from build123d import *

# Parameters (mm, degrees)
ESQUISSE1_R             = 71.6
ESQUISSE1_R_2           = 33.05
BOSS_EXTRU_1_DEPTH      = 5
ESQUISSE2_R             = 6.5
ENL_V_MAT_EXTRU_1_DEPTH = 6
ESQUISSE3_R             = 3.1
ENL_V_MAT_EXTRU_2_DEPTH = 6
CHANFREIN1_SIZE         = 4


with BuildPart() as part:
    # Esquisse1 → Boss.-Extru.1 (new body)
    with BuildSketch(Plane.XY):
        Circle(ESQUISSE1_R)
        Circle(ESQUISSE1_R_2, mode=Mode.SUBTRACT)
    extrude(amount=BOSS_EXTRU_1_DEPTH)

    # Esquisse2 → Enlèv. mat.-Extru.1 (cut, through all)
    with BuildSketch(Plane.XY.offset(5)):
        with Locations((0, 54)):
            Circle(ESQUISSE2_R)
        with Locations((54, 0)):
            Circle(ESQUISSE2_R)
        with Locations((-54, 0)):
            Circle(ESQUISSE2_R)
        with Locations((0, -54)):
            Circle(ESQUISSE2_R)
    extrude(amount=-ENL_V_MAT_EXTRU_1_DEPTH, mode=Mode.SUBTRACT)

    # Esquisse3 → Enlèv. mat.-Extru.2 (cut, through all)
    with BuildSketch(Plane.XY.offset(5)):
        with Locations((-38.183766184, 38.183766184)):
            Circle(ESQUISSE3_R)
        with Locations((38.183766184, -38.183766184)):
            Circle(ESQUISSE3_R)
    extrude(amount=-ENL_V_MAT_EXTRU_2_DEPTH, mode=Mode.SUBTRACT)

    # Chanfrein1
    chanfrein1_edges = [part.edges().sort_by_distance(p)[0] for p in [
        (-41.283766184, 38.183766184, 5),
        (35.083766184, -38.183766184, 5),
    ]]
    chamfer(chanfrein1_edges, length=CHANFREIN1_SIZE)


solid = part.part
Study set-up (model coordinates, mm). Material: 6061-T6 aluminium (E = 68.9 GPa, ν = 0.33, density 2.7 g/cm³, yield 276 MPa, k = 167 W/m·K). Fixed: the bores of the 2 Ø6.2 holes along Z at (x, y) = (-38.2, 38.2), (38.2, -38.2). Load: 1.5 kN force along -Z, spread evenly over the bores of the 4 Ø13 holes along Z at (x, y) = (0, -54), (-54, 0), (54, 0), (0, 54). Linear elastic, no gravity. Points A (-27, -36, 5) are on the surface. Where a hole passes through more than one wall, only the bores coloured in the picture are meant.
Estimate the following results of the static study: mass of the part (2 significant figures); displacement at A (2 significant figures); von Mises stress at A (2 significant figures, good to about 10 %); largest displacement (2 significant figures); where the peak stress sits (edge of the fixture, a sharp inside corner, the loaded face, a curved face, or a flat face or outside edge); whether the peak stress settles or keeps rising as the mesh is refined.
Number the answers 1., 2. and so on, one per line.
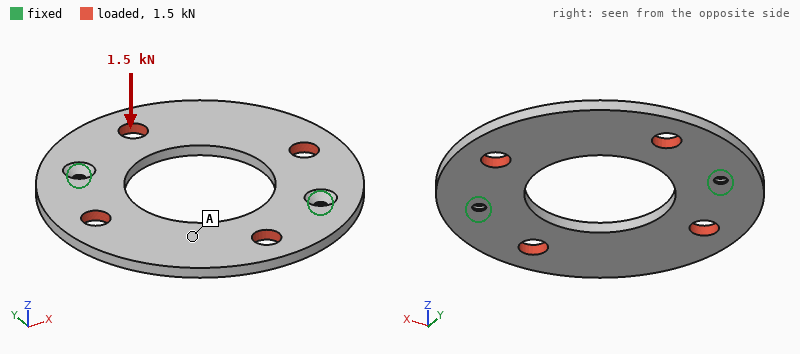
1. 160 g
2. 0.50 mm
3. 21 MPa
4. 0.79 mm
5. edge of the fixture
6. keeps rising
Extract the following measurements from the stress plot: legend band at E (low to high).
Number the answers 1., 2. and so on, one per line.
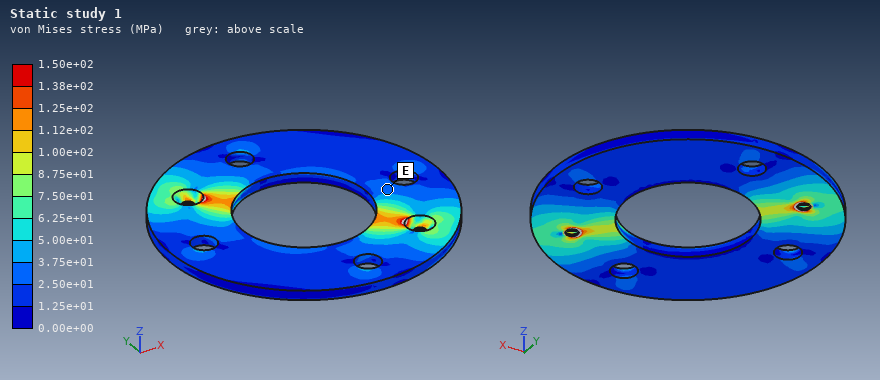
1. 2.50e+01 to 3.75e+01 MPa
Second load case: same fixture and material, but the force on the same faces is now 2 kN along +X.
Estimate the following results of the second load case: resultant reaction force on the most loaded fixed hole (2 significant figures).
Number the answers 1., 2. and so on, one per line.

1. 1.0 kN
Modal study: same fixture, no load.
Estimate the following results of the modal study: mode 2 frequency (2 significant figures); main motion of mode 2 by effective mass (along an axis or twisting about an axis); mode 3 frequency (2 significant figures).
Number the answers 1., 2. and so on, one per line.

1. 680 Hz
2. along Z
3. 1300 Hz
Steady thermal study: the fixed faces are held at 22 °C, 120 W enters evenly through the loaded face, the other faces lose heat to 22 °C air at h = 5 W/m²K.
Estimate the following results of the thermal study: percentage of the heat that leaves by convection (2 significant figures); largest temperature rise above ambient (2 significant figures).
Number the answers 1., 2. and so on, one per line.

1. 5.9 %
2. 67 K
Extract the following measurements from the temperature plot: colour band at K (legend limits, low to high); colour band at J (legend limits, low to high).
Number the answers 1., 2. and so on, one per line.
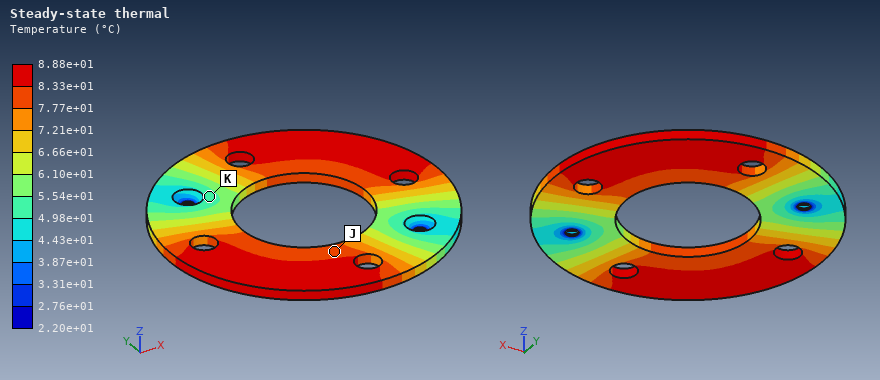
1. 4.98e+01 to 5.54e+01 °C
2. 7.77e+01 to 8.33e+01 °C
